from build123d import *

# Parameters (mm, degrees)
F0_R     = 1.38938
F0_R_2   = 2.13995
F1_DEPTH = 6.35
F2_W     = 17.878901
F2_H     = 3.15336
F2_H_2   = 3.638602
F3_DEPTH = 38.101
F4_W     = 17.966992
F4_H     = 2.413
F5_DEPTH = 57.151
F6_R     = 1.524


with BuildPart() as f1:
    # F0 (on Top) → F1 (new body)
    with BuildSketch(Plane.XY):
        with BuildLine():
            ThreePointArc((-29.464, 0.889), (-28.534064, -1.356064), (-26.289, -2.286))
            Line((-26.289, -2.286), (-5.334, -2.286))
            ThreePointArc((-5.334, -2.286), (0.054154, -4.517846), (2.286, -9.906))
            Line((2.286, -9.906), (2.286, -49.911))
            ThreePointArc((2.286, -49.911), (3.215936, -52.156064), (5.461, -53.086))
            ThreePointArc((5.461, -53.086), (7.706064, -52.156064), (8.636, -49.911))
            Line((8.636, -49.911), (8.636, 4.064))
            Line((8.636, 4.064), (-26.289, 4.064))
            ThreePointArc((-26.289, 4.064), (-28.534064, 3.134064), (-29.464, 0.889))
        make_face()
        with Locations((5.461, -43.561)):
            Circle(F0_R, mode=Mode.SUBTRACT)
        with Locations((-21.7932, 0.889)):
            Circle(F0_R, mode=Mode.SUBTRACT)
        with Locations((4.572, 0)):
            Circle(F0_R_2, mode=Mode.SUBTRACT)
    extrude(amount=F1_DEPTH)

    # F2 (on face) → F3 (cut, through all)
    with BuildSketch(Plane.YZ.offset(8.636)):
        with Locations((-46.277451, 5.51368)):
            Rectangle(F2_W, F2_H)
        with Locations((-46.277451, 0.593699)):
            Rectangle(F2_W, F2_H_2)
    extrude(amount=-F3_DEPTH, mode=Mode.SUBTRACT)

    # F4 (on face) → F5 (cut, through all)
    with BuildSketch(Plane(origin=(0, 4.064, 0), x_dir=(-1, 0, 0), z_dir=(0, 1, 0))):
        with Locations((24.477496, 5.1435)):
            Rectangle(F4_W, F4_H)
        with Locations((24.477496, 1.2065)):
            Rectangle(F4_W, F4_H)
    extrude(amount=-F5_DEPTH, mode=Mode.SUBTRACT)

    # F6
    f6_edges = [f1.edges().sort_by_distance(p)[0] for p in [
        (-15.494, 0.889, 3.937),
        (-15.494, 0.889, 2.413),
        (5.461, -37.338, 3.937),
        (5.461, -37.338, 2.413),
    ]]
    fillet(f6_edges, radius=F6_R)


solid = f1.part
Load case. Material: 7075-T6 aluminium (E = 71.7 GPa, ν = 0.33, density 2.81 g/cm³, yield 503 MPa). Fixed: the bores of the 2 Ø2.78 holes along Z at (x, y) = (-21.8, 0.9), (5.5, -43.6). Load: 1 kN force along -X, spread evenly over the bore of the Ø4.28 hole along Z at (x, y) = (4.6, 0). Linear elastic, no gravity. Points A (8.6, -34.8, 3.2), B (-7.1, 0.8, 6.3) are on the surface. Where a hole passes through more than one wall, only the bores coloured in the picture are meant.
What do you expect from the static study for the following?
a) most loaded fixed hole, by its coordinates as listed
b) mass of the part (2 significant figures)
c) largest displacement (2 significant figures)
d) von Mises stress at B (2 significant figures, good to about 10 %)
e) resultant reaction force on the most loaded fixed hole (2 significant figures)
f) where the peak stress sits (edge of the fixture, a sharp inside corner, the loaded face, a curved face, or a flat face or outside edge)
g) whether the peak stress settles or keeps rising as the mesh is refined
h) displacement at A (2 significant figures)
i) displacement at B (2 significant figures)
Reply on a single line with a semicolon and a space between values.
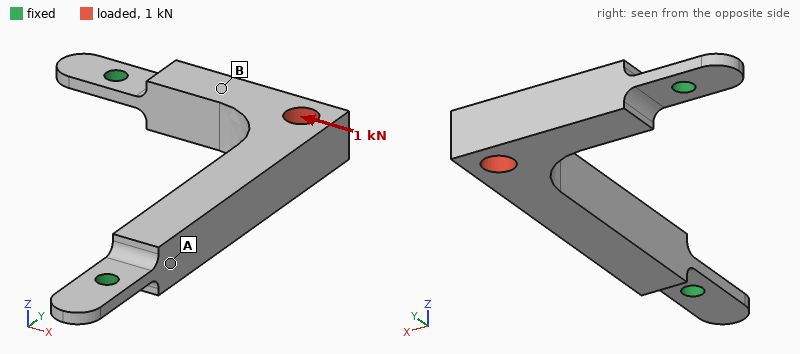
(-21.8, 0.9); 7.4 g; 18 µm; 24 MPa; 990 N; edge of the fixture; keeps rising; 3.4 µm; 12 µm
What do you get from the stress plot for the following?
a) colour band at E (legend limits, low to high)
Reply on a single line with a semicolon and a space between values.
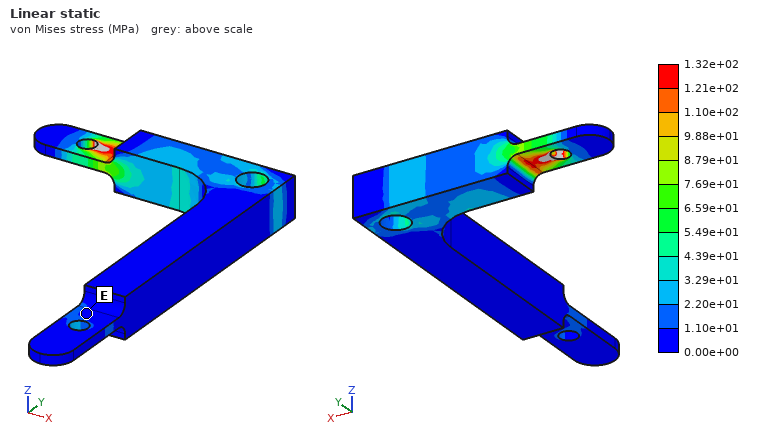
0.00e+00 to 1.10e+01 MPa
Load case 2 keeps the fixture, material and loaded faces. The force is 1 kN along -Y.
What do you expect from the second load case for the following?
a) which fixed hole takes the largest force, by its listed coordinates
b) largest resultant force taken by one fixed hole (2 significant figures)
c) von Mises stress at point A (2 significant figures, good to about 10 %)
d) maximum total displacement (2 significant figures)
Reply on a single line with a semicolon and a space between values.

(5.5, -43.6); 950 N; 39 MPa; 23 µm
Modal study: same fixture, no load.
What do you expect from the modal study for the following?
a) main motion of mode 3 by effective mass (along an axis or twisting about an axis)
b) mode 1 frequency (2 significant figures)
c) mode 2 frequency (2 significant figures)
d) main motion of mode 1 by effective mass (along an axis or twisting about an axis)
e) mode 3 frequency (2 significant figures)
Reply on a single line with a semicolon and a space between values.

along X; 1300 Hz; 9000 Hz; along Z; 11 kHz
